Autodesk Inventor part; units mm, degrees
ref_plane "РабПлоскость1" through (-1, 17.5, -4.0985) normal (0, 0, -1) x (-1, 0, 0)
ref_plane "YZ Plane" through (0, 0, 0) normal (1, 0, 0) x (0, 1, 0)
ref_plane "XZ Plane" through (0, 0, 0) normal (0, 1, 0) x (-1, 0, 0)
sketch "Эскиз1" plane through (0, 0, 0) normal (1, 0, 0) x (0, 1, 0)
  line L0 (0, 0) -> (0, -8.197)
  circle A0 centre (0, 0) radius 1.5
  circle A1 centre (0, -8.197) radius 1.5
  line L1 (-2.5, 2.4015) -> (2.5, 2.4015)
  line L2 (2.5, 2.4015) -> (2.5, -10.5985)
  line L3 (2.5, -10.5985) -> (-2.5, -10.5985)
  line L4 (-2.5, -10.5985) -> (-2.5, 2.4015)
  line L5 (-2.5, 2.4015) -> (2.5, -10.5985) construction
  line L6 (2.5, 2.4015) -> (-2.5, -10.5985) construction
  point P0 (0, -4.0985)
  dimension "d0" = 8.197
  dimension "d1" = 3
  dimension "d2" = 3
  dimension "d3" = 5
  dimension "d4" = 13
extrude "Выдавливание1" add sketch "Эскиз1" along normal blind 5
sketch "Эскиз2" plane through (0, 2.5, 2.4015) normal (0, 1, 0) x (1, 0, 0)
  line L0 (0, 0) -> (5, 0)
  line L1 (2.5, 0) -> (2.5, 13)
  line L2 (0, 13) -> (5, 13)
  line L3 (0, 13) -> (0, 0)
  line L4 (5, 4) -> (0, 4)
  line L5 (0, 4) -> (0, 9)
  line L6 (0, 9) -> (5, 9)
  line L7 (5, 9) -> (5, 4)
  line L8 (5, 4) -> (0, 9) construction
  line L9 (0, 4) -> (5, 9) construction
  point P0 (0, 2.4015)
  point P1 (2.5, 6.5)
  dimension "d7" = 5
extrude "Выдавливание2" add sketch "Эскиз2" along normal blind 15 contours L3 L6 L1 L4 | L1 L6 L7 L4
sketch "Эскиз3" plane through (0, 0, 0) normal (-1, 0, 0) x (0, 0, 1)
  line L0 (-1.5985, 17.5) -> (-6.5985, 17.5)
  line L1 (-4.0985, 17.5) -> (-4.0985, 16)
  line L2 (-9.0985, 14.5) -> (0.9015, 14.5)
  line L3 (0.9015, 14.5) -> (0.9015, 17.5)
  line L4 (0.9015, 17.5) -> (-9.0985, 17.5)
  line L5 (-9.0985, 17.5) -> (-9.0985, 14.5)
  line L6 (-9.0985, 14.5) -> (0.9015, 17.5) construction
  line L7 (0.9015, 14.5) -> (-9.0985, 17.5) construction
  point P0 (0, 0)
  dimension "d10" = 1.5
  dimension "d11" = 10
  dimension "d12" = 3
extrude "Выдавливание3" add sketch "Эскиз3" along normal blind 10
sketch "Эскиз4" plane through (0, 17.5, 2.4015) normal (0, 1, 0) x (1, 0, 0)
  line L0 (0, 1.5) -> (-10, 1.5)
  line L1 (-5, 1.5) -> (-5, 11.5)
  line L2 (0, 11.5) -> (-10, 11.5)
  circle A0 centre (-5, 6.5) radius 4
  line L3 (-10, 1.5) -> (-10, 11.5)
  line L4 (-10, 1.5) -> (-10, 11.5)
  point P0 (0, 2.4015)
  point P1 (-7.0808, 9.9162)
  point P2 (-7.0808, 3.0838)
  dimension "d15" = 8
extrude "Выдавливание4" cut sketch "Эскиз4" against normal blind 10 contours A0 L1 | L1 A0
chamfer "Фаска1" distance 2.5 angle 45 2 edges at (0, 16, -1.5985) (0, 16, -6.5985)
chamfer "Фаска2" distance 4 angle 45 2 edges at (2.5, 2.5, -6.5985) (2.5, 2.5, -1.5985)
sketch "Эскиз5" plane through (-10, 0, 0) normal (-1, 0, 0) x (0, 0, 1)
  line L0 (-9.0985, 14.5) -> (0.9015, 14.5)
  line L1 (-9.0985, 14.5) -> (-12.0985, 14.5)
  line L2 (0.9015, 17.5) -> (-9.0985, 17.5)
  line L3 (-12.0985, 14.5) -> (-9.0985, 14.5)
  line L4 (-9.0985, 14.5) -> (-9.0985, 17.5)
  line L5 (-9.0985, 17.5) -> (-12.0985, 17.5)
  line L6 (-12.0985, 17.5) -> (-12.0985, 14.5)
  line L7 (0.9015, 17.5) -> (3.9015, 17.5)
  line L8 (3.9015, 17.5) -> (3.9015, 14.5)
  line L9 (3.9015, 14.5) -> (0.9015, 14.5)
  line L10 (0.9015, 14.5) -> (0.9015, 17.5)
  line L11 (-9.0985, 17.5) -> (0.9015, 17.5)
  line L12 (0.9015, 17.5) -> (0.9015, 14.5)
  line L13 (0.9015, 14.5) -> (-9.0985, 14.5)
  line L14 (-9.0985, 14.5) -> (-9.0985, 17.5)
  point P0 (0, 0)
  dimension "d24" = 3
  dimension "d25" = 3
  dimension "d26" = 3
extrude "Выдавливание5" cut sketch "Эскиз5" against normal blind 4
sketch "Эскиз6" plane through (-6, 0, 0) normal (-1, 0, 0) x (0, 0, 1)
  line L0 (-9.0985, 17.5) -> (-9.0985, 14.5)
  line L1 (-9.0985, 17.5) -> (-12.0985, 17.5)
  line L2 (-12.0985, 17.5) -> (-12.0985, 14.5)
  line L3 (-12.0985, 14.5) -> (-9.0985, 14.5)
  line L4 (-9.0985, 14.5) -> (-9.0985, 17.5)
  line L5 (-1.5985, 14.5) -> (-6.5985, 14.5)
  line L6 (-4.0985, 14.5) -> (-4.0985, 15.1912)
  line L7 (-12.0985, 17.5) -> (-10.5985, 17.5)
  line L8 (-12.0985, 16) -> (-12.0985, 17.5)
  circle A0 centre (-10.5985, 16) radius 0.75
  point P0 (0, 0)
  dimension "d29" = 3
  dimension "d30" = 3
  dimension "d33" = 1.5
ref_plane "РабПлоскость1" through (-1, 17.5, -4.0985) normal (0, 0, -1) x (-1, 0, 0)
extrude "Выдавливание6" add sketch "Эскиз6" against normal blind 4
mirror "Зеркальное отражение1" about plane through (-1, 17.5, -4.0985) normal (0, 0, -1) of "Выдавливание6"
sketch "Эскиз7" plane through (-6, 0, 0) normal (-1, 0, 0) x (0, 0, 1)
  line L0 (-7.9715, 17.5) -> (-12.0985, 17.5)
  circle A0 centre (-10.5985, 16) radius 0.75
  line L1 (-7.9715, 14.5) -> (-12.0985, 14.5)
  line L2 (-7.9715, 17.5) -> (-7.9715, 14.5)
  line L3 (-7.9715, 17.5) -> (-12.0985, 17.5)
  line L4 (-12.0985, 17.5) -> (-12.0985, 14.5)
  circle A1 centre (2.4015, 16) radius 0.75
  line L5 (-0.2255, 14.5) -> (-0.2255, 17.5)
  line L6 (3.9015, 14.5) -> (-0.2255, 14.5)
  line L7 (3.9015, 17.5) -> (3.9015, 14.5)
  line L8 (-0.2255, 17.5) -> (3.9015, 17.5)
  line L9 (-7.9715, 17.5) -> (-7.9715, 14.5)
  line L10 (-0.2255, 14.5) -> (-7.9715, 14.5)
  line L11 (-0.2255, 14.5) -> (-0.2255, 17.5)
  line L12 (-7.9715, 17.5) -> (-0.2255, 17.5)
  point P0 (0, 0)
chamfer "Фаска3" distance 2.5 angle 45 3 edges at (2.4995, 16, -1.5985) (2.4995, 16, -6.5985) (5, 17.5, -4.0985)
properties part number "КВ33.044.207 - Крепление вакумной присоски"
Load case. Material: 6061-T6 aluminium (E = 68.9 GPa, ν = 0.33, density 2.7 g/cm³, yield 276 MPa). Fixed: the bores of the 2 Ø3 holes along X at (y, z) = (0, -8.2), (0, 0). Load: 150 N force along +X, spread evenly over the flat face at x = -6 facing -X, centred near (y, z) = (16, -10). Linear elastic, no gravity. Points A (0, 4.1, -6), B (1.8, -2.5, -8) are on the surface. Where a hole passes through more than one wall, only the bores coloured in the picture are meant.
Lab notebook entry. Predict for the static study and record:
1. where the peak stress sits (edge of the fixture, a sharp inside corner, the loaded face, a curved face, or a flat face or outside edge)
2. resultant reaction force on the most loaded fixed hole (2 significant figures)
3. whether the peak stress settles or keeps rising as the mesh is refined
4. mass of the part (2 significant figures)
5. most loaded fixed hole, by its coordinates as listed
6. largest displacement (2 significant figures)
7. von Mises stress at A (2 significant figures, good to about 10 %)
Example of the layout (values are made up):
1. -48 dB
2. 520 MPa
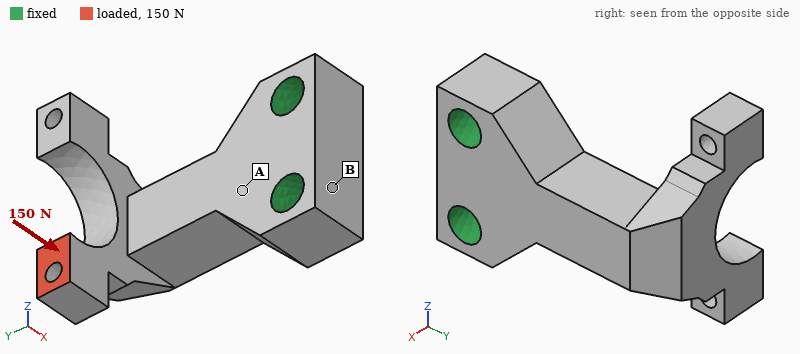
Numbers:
1. a sharp inside corner
2. 170 N
3. keeps rising
4. 2.3 g
5. (0, -8.2)
6. 0.13 mm
7. 62 MPa
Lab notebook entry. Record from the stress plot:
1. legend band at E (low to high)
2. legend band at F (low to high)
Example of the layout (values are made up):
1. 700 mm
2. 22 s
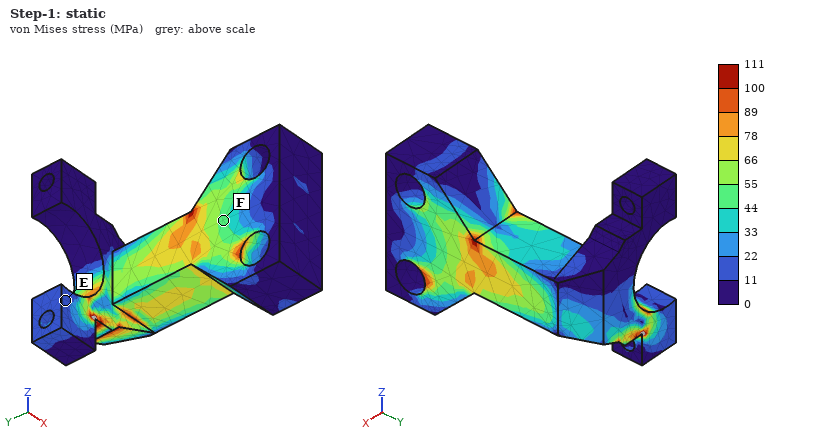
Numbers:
1. 11 to 22 MPa
2. 44 to 55 MPa
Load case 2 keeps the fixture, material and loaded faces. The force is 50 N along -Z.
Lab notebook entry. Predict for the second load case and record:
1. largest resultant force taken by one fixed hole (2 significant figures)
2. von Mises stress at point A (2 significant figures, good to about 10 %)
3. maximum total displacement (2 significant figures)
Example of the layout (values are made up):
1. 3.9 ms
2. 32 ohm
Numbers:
1. 100 N
2. 9.1 MPa
3. 59 µm
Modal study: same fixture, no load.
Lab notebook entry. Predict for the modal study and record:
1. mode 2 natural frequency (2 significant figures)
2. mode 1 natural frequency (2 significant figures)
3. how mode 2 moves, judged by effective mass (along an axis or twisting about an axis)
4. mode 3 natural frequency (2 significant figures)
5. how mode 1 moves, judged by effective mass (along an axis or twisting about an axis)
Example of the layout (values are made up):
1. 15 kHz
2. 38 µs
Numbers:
1. 11 kHz
2. 10 kHz
3. along Z
4. 17 kHz
5. along X
